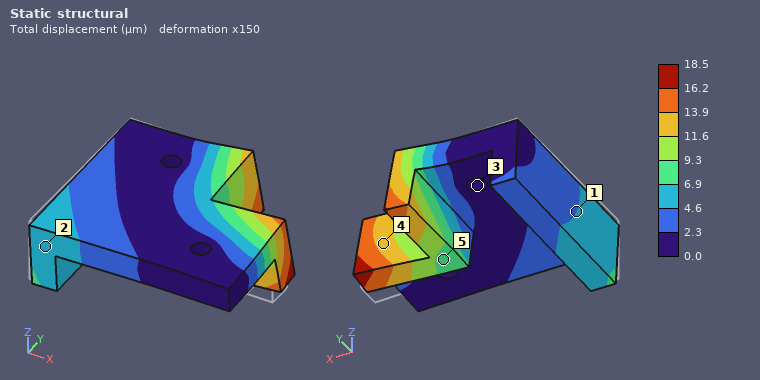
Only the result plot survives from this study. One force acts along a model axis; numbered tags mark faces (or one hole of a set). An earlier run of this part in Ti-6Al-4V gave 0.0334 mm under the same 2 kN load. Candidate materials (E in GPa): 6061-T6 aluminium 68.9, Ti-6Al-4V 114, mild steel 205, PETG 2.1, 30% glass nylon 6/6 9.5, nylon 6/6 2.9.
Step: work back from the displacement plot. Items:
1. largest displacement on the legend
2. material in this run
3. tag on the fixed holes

18.5 µm
mild steel
3
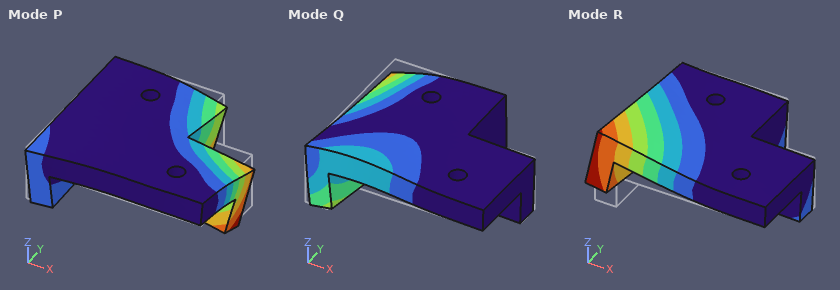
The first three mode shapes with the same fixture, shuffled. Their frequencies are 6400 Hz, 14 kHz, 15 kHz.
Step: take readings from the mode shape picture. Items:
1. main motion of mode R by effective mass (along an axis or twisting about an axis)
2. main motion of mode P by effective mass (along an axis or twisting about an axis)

along Z
along Z
